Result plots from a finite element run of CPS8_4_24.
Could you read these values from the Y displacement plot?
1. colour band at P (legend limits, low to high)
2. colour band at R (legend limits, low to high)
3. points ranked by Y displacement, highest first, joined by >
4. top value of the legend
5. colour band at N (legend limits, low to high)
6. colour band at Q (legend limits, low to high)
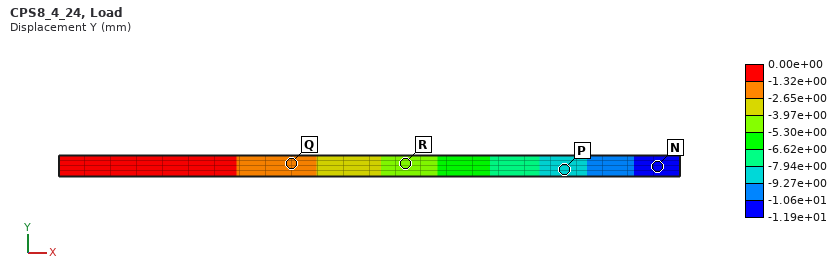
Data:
-9.27e+00 to -7.94e+00 mm
-5.30e+00 to -3.97e+00 mm
Q > R > P > N
0.00e+00 mm
-1.19e+01 to -1.06e+01 mm
-2.65e+00 to -1.32e+00 mm
